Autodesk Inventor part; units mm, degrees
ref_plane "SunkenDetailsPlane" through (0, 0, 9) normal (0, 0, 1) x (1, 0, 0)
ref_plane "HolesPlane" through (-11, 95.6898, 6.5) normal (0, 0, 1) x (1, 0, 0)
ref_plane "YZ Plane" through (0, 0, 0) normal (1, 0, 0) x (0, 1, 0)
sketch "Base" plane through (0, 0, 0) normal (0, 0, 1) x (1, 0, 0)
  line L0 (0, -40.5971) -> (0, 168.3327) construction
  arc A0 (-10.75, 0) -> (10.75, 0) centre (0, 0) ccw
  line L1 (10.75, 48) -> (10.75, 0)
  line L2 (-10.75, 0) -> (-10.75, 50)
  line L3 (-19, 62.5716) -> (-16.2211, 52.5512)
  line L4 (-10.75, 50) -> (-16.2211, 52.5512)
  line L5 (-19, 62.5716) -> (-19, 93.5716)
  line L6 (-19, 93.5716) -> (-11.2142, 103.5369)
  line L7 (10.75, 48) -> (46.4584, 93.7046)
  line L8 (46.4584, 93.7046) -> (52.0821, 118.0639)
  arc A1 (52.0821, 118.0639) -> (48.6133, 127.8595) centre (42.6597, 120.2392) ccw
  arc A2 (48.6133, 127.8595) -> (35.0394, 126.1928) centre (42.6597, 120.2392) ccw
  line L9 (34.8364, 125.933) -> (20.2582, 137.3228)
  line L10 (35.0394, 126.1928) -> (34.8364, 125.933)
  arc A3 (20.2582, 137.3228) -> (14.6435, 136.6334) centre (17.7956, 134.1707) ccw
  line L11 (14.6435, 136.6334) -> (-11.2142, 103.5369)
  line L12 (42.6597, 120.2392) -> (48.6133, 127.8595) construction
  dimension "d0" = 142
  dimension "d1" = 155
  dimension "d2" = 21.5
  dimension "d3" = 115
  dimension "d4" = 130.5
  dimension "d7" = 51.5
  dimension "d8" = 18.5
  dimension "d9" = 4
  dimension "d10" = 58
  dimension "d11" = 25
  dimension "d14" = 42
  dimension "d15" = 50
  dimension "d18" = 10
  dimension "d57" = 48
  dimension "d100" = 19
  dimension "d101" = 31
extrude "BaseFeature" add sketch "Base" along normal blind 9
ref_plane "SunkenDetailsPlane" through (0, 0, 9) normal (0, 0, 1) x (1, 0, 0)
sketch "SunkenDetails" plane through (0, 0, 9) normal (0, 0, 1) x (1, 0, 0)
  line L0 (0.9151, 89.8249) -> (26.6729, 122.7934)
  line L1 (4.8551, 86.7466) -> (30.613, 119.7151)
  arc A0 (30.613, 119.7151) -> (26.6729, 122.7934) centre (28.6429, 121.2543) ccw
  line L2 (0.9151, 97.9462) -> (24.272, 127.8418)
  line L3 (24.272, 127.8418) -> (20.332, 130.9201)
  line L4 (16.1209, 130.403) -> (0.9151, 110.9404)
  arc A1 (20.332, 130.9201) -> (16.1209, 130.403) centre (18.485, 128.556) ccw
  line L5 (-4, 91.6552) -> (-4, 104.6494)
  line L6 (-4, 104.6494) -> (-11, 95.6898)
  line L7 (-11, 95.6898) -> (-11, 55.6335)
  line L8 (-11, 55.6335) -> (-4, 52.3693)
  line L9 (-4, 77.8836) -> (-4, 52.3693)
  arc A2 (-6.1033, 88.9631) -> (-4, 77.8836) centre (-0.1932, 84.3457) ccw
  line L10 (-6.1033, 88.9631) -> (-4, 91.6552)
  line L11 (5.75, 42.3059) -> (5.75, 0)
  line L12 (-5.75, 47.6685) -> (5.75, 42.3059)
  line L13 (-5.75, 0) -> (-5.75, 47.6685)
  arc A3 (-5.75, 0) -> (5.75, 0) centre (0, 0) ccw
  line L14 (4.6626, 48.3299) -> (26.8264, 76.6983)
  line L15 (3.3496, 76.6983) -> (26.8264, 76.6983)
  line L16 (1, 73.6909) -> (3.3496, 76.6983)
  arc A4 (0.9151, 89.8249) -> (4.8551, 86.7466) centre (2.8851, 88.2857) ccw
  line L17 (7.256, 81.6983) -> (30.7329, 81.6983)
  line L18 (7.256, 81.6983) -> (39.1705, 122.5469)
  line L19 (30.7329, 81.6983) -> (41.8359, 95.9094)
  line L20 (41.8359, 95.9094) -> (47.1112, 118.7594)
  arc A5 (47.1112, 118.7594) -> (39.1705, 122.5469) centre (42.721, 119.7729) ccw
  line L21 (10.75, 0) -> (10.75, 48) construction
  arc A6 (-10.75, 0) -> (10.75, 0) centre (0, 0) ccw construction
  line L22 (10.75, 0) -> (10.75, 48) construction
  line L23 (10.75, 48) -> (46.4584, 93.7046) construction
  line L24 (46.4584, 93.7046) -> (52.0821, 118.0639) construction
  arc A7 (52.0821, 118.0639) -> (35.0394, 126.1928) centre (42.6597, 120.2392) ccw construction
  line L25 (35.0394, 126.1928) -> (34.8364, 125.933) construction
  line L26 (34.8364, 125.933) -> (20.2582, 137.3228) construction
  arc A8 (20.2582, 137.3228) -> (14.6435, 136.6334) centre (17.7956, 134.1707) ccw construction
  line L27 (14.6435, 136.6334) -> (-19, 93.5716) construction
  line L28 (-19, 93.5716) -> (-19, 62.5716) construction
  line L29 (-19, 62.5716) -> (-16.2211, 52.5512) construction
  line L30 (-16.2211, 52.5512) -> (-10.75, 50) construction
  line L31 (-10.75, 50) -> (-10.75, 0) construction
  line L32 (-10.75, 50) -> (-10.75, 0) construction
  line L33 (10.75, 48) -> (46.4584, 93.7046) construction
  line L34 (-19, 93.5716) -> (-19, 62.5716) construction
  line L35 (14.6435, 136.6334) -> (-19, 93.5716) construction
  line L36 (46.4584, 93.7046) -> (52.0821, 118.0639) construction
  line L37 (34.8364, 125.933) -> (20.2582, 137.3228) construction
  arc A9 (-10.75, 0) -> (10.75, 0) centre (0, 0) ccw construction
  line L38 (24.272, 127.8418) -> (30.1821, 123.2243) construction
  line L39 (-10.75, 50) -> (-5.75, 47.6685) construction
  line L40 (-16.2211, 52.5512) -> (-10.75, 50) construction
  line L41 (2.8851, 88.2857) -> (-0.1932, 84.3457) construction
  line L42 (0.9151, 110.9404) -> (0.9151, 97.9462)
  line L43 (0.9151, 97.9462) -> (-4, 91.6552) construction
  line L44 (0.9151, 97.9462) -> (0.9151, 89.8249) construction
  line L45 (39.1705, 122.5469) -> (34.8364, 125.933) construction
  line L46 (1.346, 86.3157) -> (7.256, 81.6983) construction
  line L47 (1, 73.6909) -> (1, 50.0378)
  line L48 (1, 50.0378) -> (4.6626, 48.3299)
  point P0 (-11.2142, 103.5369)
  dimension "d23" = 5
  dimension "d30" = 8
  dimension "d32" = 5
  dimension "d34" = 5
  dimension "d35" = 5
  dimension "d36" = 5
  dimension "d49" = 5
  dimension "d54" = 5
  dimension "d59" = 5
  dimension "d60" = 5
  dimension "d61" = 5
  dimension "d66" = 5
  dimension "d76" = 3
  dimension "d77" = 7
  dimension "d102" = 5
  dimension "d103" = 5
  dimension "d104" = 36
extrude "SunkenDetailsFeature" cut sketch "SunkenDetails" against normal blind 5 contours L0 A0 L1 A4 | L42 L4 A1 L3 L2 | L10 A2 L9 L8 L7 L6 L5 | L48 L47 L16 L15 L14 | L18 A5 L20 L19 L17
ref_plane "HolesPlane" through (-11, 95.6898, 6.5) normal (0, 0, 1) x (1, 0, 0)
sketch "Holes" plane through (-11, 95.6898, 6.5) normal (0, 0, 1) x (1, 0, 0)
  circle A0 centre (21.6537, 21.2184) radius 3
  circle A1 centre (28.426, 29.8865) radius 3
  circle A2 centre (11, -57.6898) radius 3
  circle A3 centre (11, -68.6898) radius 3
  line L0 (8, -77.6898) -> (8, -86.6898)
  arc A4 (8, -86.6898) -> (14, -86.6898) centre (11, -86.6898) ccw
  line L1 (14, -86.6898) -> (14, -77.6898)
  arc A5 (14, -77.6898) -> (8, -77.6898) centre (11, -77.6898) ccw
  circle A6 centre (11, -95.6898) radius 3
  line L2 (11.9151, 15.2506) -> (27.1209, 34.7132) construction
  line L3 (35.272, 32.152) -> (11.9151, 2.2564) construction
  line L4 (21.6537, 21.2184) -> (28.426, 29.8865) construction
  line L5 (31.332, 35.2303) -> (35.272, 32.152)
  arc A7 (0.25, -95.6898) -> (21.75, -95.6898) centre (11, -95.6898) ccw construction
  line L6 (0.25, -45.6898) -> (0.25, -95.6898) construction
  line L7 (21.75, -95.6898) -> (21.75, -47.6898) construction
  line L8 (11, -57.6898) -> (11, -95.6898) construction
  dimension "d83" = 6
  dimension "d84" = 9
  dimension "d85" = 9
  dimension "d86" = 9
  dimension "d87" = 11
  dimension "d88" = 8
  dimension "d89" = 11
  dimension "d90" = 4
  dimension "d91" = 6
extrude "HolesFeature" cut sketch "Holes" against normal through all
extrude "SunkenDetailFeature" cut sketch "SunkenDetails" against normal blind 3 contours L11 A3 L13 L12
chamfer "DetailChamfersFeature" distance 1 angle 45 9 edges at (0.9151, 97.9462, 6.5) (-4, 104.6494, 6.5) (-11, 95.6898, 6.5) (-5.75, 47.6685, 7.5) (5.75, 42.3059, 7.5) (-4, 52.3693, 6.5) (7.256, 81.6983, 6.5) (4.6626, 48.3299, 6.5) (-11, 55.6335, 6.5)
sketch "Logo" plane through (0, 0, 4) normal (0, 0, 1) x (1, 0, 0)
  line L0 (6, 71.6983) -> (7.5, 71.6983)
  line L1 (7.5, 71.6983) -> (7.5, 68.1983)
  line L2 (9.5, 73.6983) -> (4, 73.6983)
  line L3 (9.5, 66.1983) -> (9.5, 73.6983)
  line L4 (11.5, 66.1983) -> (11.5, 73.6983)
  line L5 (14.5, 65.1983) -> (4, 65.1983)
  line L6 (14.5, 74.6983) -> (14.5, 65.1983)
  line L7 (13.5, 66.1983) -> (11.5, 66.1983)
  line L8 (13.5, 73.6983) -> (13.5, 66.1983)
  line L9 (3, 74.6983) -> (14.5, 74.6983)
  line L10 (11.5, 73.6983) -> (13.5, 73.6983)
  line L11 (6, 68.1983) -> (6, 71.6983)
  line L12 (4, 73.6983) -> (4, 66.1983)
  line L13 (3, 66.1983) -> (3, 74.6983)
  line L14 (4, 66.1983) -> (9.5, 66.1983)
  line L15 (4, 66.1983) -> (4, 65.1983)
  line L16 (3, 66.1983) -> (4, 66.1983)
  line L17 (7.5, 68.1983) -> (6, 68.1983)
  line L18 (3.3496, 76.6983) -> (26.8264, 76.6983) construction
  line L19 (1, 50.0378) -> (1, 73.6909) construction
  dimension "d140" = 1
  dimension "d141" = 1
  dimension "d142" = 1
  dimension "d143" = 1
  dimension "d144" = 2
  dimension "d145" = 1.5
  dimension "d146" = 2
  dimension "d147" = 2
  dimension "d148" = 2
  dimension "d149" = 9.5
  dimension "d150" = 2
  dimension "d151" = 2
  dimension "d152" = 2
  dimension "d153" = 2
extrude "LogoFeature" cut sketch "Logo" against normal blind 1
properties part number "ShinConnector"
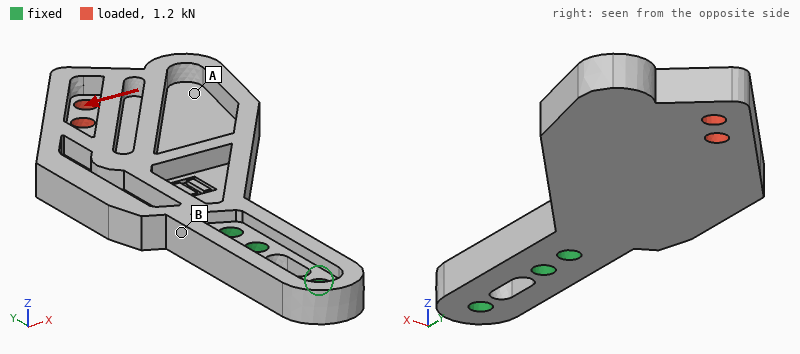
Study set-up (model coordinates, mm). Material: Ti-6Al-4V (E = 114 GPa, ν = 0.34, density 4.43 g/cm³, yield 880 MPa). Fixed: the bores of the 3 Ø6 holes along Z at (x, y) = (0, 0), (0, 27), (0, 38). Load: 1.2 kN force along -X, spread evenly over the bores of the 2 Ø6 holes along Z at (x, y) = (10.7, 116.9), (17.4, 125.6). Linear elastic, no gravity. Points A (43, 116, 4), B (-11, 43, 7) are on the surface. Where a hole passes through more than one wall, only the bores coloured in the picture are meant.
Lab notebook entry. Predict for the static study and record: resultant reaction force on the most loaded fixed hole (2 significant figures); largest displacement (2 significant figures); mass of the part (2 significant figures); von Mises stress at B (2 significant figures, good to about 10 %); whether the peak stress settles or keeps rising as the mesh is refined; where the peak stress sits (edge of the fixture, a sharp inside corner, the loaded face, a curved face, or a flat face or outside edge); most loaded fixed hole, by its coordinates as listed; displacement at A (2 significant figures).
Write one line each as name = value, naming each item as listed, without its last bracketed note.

resultant reaction force on the most loaded fixed hole = 4.8 kN
largest displacement = 0.40 mm
mass of the part = 160 g
von Mises stress at B = 130 MPa
whether the peak stress settles or keeps rising as the mesh is refined = keeps rising
where the peak stress sits = edge of the fixture
most loaded fixed hole, by its coordinates as listed = (0, 38)
displacement at A = 0.34 mm
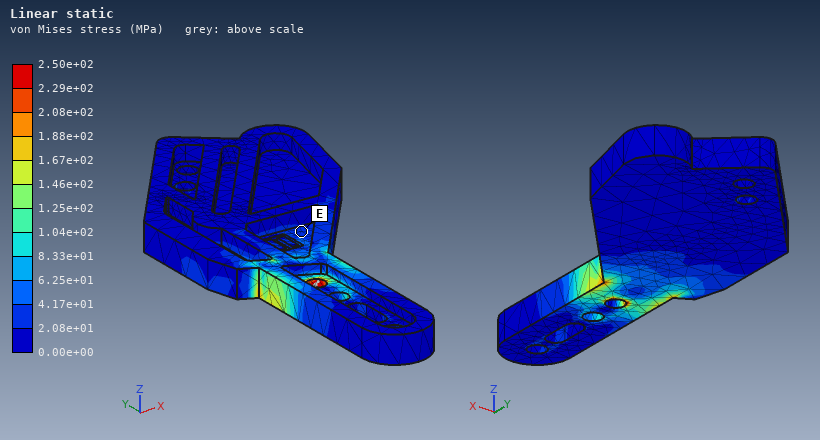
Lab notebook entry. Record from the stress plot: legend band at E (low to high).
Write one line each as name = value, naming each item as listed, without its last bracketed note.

legend band at E = 2.08e+01 to 4.17e+01 MPa
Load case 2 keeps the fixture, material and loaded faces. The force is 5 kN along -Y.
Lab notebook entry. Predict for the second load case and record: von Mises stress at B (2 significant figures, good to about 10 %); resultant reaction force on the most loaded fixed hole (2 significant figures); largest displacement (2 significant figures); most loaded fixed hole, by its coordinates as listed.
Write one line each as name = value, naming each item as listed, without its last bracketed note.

von Mises stress at B = 99 MPa
resultant reaction force on the most loaded fixed hole = 4.8 kN
largest displacement = 0.40 mm
most loaded fixed hole, by its coordinates as listed = (0, 38)
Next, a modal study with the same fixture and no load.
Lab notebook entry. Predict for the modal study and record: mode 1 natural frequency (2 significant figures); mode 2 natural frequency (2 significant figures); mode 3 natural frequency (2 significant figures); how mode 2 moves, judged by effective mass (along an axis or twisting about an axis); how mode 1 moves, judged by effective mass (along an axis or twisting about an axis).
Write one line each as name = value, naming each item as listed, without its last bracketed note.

mode 1 natural frequency = 520 Hz
mode 2 natural frequency = 1200 Hz
mode 3 natural frequency = 1500 Hz
how mode 2 moves, judged by effective mass = along X
how mode 1 moves, judged by effective mass = along Z
